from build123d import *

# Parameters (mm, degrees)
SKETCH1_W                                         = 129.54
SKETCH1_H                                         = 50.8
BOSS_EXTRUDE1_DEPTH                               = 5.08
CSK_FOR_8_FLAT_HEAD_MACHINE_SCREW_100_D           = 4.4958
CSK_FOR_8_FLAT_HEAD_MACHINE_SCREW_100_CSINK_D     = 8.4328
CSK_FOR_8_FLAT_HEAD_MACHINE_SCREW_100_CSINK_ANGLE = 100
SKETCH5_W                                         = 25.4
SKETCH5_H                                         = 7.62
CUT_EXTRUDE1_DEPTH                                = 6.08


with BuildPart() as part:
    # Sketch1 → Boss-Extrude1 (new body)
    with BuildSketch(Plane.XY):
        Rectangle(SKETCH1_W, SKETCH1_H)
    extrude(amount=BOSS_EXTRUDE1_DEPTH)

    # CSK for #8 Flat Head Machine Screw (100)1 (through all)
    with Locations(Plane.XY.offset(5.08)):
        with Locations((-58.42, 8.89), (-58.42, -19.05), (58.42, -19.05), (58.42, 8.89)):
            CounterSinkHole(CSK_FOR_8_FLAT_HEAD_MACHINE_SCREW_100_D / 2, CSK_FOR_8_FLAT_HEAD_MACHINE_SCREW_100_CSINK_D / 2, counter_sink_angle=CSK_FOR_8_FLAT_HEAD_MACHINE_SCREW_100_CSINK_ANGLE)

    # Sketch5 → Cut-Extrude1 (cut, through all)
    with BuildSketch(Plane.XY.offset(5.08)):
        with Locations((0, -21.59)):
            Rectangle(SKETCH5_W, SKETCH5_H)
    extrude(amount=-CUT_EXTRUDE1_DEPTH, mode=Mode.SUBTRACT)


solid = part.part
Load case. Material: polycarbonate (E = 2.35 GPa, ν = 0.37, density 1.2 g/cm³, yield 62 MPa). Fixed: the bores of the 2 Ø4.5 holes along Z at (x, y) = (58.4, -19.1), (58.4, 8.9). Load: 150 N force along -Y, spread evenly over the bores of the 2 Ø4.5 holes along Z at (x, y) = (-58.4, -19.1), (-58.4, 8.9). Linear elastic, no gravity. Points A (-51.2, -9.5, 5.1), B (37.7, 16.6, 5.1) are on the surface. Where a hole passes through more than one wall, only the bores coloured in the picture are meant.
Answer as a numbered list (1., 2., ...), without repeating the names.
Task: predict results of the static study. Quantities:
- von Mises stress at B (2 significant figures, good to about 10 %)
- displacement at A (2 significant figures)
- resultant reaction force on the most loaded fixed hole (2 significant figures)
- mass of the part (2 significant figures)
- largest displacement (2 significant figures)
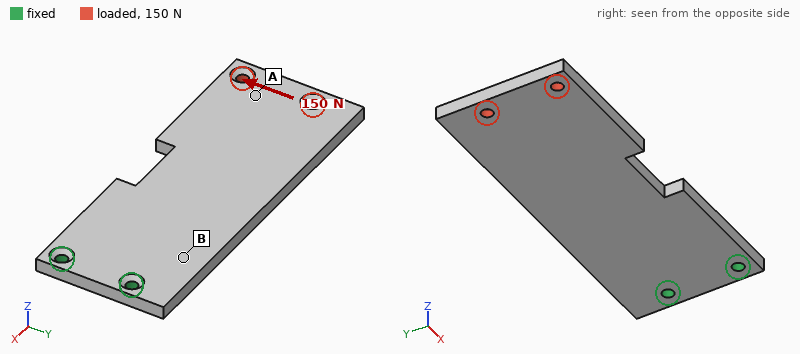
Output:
1. 4.5 MPa
2. 0.97 mm
3. 590 N
4. 38 g
5. 1.3 mm
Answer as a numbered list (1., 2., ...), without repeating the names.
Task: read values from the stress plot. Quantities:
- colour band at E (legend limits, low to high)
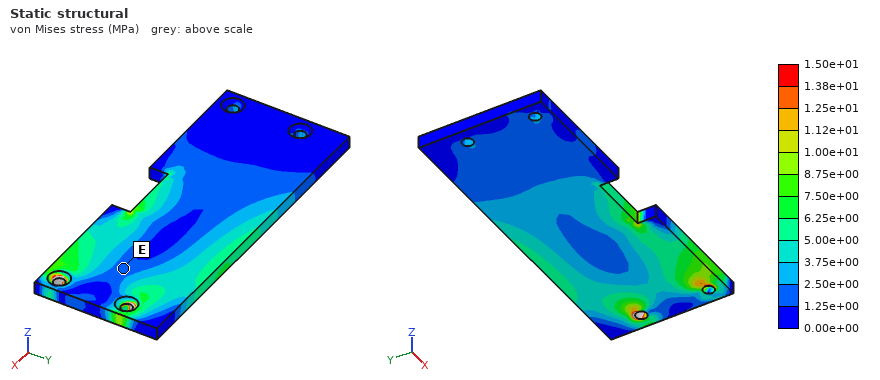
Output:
1. 1.25e+00 to 2.50e+00 MPa
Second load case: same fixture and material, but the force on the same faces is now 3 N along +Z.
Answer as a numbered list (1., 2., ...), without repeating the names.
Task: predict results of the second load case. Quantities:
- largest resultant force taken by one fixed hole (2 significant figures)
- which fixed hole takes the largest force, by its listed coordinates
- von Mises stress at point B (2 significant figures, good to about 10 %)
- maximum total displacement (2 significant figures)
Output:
1. 2.5 N
2. (58.4, 8.9)
3. 1.3 MPa
4. 1.5 mm
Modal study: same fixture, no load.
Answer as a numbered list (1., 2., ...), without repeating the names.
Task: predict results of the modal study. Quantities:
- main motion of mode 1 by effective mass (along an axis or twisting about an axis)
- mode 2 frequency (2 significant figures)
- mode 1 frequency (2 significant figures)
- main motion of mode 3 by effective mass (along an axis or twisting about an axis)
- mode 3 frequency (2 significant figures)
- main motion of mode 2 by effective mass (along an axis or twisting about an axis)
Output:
1. along Z
2. 350 Hz
3. 72 Hz
4. along Z
5. 450 Hz
6. twisting about X
